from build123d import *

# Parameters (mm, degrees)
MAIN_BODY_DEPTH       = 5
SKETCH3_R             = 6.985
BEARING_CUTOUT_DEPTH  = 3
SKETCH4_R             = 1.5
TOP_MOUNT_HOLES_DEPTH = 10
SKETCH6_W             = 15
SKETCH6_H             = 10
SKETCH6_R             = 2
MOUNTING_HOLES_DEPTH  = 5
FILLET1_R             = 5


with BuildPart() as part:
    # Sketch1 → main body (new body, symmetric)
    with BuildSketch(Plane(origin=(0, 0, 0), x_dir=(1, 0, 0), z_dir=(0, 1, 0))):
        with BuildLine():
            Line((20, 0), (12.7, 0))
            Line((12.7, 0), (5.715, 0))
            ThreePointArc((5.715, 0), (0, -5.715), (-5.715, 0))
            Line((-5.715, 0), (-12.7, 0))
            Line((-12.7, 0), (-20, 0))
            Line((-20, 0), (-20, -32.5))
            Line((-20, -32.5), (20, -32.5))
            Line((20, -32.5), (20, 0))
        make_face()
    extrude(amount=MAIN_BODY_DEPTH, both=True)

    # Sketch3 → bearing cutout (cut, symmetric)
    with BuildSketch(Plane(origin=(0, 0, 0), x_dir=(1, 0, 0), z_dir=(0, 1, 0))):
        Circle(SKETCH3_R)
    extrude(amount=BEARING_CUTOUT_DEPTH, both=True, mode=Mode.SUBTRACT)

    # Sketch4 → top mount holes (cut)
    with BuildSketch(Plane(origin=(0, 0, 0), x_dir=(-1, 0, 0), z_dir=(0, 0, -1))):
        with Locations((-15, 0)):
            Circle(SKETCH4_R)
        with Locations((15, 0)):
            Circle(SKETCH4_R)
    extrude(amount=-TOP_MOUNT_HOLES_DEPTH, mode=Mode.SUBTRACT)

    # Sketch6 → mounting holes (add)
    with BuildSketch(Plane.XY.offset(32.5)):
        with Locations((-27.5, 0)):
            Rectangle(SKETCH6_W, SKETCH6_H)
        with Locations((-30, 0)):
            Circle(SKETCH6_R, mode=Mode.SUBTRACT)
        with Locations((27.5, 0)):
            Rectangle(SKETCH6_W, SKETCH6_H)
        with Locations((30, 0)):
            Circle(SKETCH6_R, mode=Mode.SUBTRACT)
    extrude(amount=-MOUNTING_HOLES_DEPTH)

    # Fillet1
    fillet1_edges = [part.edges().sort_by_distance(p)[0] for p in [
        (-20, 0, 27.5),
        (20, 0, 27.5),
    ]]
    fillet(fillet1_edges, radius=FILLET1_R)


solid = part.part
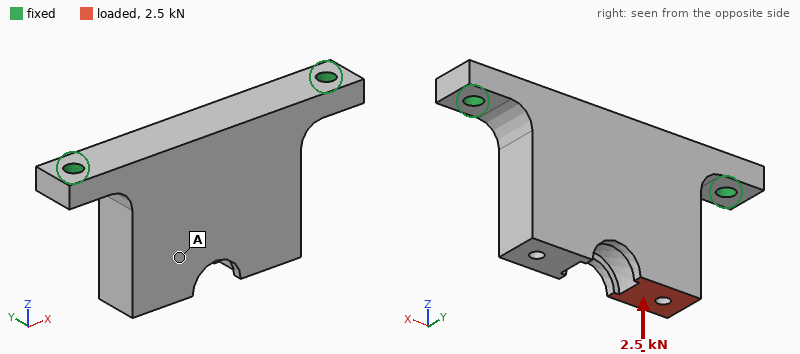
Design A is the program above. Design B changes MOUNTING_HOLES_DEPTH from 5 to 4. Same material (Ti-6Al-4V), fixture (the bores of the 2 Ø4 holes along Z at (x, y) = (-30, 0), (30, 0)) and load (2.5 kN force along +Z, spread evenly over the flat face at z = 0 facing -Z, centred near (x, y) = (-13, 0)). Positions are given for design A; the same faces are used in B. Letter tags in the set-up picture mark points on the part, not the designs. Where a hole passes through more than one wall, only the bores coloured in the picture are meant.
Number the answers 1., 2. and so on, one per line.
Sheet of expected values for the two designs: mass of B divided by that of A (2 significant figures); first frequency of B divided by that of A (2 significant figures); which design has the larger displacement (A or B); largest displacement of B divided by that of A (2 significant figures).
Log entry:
1. 0.98
2. 0.80
3. B
4. 1.3
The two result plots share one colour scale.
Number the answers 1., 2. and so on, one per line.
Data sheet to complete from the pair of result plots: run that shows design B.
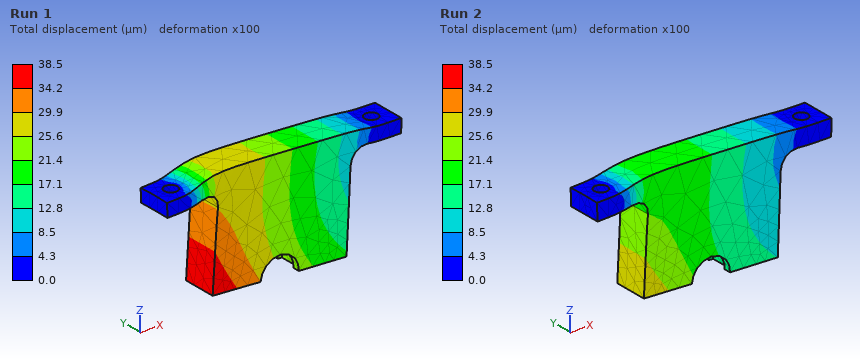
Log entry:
1. Run 1
